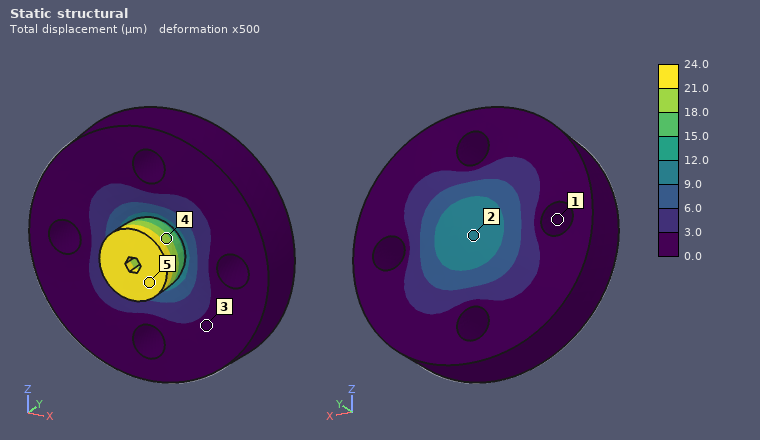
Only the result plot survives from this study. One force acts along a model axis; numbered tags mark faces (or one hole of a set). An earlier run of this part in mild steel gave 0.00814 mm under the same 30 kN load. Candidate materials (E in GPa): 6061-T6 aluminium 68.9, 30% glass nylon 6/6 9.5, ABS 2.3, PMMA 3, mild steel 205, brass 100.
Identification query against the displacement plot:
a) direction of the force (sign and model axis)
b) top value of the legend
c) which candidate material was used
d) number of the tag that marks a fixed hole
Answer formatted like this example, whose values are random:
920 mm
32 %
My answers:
+Y
24.0 µm
6061-T6 aluminium
1
